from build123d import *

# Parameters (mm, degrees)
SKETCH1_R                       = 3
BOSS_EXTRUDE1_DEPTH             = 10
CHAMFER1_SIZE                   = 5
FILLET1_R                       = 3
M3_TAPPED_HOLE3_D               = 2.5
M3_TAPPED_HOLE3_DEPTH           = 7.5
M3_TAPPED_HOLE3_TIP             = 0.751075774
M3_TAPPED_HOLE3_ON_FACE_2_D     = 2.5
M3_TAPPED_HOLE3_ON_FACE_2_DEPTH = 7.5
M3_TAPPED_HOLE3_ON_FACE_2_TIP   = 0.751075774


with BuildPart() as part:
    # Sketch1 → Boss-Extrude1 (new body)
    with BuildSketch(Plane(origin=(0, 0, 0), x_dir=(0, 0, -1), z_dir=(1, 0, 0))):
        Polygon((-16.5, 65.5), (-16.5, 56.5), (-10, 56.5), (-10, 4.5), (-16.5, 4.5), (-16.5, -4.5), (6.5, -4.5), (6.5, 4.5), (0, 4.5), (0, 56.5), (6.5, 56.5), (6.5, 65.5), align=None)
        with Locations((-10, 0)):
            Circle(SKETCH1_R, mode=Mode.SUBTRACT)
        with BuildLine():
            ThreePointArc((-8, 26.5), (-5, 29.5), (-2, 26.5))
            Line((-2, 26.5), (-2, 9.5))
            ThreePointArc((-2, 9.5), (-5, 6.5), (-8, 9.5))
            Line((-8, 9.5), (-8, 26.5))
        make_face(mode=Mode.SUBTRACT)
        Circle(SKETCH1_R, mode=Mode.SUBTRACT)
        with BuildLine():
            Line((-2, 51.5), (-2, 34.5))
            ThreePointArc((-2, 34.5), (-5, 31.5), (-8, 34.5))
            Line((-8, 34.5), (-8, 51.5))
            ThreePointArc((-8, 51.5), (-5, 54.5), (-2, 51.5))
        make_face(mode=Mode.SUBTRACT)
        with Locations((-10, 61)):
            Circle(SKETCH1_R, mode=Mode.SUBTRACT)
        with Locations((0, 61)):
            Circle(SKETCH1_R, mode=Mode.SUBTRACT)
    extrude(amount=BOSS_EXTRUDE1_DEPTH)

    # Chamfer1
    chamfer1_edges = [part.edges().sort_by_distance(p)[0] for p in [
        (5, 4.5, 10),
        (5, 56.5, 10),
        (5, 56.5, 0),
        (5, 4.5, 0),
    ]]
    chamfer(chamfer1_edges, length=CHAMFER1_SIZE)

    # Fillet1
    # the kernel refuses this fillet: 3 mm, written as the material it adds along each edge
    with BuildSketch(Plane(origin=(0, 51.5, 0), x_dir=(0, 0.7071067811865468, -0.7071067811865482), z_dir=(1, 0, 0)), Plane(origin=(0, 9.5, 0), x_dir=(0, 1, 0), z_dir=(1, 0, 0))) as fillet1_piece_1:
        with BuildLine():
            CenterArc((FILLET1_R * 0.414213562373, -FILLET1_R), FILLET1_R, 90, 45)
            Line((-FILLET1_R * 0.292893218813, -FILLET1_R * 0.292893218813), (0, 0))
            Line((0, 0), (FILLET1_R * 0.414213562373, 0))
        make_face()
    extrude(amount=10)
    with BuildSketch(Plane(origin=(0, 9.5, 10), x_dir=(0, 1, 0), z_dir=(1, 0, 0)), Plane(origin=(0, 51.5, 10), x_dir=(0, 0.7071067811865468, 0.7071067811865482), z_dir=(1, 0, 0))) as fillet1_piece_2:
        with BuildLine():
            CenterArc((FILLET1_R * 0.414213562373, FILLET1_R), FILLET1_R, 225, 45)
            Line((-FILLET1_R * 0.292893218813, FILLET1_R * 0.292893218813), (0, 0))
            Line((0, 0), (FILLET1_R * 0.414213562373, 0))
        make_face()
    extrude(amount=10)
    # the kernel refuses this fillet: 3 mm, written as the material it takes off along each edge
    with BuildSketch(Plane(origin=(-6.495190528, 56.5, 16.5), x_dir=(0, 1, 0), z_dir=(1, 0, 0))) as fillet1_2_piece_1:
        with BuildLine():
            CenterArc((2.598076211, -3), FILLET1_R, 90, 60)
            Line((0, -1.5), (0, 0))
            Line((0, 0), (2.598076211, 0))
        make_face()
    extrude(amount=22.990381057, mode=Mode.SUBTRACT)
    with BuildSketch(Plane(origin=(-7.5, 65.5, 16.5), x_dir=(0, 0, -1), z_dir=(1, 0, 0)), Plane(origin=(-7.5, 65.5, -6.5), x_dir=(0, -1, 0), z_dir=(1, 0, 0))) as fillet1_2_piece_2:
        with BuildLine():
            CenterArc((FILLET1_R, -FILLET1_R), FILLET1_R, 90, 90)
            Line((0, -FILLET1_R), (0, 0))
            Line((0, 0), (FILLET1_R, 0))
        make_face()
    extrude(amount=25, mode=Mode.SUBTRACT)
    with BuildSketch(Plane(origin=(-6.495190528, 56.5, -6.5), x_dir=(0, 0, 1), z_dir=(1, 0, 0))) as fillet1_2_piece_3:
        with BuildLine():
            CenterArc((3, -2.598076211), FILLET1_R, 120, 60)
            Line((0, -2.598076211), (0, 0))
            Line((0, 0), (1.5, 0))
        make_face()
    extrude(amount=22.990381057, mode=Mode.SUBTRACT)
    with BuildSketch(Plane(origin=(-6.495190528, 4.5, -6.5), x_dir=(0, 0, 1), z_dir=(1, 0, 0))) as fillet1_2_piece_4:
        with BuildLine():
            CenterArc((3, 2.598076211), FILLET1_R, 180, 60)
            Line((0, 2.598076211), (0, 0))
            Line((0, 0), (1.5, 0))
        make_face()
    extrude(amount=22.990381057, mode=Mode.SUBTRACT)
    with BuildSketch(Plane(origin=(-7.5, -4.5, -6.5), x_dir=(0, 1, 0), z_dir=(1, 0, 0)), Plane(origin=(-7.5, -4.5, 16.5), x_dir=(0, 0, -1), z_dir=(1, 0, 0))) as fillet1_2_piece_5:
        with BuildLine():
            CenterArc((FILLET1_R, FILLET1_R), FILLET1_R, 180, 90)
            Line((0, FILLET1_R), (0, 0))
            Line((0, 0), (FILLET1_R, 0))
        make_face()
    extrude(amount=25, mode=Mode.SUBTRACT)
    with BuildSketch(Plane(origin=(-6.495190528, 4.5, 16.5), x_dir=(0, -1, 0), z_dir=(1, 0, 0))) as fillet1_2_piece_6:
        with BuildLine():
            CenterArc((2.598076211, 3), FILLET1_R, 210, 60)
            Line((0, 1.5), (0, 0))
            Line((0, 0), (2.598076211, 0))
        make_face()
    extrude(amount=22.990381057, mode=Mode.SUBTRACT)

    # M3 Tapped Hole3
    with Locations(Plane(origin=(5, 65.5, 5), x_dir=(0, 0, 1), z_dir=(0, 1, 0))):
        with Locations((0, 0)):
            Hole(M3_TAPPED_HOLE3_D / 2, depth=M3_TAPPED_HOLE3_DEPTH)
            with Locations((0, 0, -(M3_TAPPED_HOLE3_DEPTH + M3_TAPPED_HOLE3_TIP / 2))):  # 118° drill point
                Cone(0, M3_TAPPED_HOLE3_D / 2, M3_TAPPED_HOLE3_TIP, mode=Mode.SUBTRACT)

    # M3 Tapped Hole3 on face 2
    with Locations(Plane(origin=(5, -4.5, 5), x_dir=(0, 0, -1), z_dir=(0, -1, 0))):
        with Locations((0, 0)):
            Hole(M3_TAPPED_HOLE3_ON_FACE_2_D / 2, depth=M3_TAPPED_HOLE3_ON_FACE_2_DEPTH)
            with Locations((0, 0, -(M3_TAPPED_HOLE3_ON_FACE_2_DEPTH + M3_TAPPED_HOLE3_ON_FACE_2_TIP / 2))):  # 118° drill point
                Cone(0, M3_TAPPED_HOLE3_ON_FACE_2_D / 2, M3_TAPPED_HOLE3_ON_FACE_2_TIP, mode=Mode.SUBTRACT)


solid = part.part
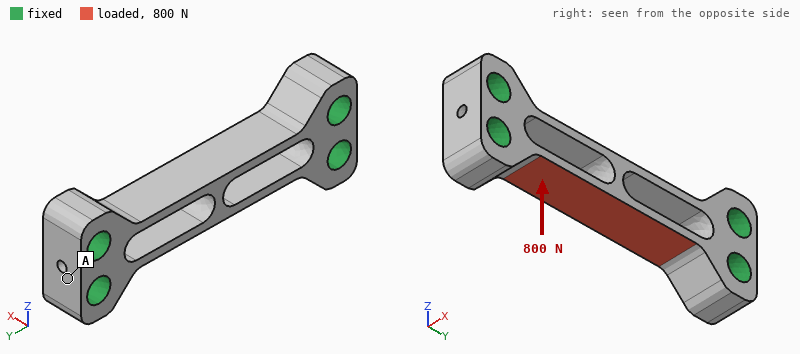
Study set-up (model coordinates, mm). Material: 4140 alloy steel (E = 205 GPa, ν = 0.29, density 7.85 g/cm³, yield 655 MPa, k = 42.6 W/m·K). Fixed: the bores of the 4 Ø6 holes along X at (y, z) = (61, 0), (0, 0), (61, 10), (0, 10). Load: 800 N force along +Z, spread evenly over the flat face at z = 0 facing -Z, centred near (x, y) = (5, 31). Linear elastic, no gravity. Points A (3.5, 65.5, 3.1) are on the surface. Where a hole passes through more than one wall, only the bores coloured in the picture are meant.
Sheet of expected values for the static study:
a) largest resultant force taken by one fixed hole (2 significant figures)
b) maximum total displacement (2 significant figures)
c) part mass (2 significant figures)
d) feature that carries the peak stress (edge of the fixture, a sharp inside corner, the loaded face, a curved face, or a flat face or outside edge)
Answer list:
460 N
60 µm
46 g
a curved face
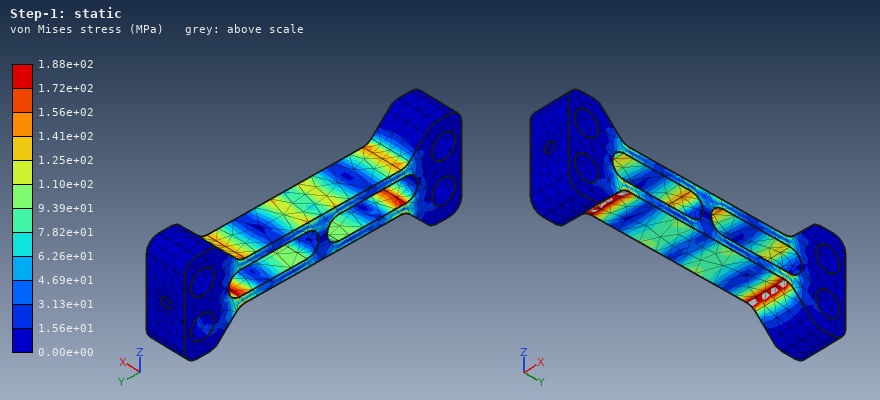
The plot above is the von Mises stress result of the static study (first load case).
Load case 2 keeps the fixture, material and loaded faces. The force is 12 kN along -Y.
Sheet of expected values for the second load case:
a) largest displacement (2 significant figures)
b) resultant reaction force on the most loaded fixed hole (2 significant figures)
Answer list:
24 µm
5.0 kN
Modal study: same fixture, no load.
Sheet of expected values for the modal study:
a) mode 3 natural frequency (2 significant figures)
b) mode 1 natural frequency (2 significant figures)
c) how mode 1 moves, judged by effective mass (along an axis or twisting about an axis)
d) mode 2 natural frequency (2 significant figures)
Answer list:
16 kHz
5200 Hz
along Z
16 kHz
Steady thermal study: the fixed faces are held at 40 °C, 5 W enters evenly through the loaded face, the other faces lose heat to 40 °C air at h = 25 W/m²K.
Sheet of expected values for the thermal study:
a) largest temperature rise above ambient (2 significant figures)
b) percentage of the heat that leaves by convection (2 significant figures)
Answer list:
23 K
11 %
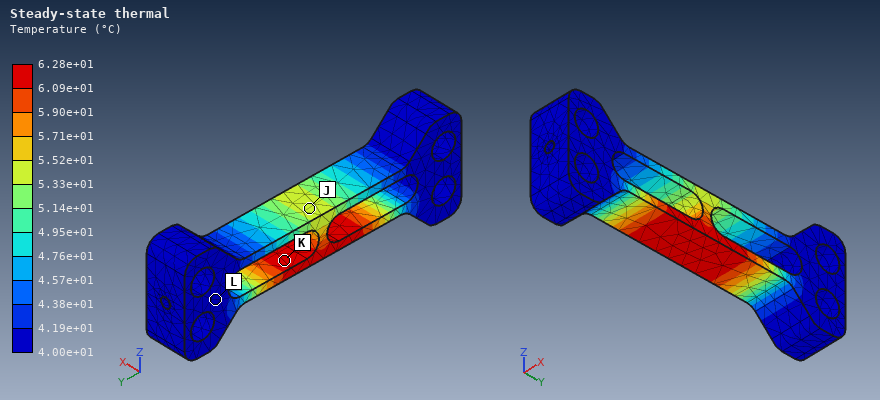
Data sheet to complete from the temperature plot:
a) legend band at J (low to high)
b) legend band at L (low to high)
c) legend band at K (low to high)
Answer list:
5.33e+01 to 5.52e+01 °C
4.00e+01 to 4.19e+01 °C
6.09e+01 to 6.28e+01 °C
